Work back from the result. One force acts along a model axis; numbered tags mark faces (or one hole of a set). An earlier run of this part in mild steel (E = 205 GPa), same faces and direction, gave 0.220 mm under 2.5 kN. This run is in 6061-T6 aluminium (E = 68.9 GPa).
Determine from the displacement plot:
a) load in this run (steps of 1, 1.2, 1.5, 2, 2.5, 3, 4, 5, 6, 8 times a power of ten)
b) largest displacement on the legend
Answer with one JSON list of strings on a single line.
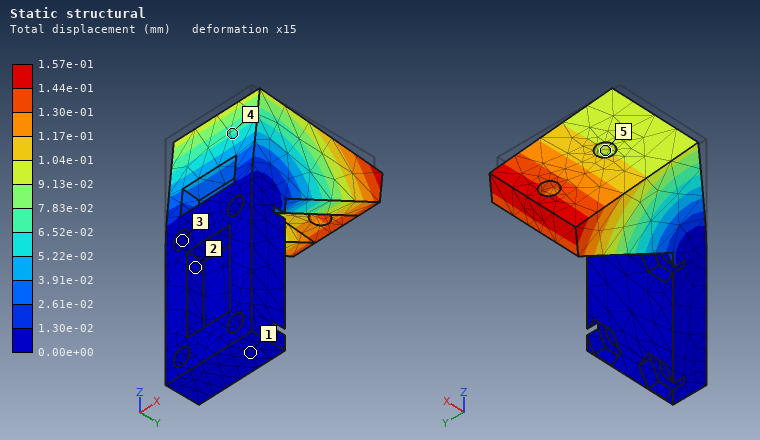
["600 N", "1.57e-01 mm"]
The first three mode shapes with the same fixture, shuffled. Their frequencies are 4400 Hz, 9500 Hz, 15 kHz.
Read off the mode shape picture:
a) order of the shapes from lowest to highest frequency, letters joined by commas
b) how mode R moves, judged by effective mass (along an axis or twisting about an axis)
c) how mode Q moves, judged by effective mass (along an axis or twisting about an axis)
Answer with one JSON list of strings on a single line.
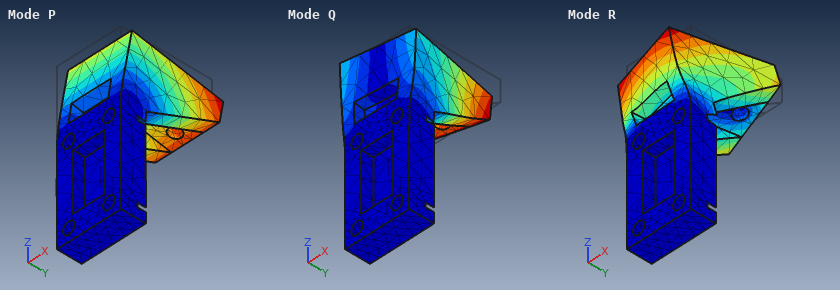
["P, Q, R", "along X", "along X"]
